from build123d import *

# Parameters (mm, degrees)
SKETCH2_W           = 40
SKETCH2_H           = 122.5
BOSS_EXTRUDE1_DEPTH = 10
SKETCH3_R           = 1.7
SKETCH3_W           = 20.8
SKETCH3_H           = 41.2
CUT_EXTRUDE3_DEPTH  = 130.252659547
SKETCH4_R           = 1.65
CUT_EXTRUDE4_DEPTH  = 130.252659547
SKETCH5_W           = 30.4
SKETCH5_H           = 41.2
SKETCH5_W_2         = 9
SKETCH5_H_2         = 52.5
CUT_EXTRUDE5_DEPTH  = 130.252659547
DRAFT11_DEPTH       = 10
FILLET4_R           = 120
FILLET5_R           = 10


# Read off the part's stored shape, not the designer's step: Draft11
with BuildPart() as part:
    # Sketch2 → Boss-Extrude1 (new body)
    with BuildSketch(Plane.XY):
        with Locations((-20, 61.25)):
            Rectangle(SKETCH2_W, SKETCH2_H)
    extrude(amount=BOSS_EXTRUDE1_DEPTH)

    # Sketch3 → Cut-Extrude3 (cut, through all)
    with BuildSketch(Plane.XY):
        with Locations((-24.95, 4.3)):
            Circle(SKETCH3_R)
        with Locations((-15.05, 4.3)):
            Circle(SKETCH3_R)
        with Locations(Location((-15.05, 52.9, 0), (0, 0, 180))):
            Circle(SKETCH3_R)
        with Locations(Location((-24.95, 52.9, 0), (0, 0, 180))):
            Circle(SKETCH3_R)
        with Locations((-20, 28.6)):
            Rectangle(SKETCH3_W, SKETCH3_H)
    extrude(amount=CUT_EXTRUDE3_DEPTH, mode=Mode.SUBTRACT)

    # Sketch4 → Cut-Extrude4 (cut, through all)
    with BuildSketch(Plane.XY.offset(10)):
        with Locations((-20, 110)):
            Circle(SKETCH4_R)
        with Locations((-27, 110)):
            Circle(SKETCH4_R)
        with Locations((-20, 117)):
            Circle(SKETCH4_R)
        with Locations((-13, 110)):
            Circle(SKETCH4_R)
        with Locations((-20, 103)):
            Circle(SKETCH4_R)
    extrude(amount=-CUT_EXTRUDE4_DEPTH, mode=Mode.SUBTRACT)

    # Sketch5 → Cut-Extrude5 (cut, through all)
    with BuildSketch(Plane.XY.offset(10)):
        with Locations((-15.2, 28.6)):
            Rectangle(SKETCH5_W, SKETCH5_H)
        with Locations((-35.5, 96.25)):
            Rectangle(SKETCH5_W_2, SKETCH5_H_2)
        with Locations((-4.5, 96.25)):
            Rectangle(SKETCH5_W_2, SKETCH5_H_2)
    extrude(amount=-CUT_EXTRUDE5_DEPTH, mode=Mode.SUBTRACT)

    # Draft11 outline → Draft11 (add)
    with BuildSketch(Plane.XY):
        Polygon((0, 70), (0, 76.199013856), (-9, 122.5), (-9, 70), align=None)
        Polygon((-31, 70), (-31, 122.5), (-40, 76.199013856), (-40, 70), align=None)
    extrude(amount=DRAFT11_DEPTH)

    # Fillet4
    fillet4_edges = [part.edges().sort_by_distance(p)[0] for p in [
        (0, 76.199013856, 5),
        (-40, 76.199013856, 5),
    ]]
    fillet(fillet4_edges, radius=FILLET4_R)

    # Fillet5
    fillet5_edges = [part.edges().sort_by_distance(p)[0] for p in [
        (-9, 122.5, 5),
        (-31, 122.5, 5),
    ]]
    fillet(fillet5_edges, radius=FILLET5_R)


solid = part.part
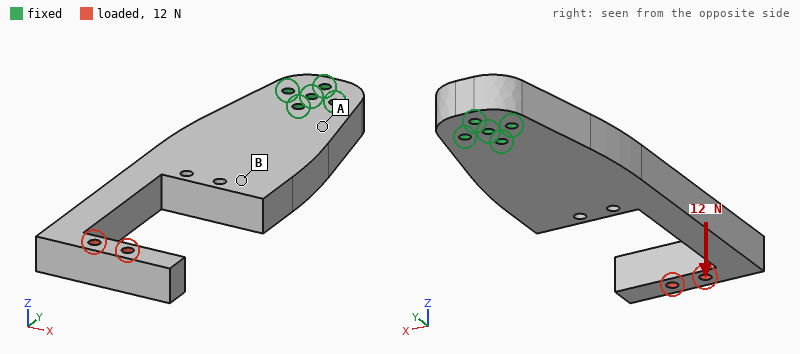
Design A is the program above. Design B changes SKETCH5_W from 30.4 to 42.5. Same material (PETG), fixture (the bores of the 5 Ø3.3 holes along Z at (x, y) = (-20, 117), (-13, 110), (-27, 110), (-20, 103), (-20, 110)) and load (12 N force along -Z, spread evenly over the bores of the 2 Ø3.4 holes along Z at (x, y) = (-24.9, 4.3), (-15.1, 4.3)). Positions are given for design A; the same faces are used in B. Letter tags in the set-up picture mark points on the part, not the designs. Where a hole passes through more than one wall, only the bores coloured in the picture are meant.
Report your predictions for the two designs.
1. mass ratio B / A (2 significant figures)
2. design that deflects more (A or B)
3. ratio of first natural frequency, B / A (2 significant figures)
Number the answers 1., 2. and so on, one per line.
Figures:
1. 0.92
2. B
3. 0.45
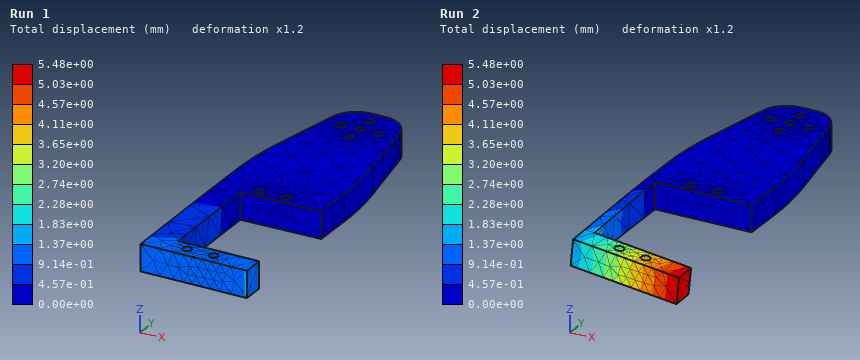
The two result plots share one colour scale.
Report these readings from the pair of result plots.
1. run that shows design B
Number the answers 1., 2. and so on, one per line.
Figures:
1. Run 2
